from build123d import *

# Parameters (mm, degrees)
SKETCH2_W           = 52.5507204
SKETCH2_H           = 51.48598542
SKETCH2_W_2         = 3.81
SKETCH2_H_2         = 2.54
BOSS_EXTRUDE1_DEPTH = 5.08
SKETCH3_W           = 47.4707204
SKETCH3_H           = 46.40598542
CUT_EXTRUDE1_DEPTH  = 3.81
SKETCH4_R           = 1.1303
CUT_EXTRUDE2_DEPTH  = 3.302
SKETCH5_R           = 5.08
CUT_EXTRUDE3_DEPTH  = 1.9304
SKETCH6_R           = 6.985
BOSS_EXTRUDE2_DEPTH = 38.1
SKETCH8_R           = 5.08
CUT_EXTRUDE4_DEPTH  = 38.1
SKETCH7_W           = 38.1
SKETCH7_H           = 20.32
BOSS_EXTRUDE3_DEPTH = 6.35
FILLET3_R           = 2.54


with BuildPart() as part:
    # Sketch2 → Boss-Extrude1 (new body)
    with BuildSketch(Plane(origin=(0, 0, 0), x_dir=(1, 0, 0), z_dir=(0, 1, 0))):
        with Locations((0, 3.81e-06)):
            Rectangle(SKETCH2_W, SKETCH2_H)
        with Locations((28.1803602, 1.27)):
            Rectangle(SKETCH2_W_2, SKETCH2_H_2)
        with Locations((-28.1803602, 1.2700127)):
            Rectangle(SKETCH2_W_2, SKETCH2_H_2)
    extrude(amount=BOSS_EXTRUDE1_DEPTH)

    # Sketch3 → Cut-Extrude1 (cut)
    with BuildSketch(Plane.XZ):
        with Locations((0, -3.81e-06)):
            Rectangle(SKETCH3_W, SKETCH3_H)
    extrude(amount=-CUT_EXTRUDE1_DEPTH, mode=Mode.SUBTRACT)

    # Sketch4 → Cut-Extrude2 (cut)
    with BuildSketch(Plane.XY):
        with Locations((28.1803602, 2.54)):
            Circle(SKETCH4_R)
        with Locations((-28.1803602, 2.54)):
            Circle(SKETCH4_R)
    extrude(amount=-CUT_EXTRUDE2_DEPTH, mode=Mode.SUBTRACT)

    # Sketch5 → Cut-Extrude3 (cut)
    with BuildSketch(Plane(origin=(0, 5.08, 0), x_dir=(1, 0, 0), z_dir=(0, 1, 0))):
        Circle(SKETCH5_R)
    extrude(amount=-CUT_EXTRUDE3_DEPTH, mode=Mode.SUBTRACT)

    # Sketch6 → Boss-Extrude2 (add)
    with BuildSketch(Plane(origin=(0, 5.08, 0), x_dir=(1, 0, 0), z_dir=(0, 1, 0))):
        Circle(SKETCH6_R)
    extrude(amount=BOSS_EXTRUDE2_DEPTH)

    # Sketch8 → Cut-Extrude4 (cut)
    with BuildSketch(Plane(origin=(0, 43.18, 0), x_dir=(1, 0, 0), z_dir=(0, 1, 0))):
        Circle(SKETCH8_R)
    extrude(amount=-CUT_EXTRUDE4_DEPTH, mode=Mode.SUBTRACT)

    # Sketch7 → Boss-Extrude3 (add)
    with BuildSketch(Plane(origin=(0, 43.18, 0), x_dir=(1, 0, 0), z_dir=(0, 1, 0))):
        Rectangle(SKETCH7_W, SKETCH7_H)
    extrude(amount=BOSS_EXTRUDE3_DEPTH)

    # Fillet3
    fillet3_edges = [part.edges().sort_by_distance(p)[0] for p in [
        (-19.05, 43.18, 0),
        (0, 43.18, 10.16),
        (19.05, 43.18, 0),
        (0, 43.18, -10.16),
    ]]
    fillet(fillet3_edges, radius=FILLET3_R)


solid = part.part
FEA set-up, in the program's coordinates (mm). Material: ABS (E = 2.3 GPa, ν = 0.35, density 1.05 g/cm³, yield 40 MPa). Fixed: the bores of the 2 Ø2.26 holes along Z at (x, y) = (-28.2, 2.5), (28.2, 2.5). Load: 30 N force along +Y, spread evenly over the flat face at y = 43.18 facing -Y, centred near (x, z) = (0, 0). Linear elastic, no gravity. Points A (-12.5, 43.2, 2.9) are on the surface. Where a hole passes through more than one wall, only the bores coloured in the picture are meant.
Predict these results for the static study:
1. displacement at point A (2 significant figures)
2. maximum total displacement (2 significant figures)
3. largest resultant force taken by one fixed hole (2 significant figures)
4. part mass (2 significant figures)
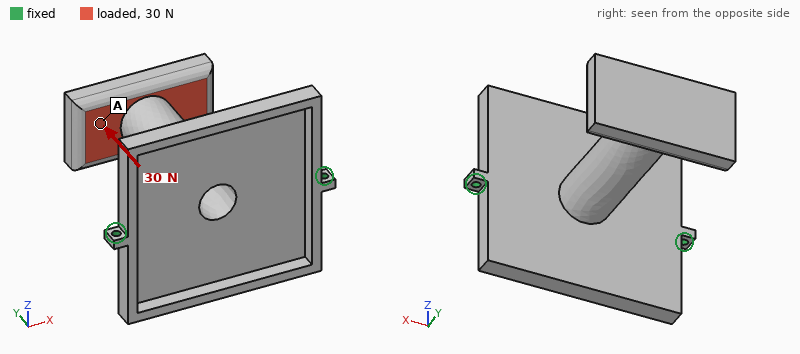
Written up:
0.63 mm
0.66 mm
27 N
13 g
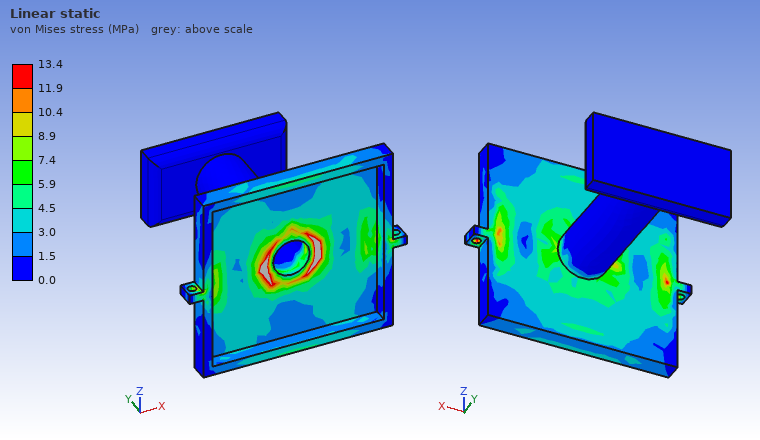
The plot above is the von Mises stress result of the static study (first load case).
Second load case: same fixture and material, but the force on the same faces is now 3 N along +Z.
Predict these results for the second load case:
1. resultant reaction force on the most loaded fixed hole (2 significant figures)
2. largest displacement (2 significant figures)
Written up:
1.5 N
1.0 mm
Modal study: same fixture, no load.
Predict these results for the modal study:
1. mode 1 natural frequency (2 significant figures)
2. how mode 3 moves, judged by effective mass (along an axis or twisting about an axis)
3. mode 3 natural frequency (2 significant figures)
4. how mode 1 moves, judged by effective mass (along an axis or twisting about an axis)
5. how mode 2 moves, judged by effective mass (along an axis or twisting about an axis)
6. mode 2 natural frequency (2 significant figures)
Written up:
110 Hz
along Y
370 Hz
along Z
along X
150 Hz
